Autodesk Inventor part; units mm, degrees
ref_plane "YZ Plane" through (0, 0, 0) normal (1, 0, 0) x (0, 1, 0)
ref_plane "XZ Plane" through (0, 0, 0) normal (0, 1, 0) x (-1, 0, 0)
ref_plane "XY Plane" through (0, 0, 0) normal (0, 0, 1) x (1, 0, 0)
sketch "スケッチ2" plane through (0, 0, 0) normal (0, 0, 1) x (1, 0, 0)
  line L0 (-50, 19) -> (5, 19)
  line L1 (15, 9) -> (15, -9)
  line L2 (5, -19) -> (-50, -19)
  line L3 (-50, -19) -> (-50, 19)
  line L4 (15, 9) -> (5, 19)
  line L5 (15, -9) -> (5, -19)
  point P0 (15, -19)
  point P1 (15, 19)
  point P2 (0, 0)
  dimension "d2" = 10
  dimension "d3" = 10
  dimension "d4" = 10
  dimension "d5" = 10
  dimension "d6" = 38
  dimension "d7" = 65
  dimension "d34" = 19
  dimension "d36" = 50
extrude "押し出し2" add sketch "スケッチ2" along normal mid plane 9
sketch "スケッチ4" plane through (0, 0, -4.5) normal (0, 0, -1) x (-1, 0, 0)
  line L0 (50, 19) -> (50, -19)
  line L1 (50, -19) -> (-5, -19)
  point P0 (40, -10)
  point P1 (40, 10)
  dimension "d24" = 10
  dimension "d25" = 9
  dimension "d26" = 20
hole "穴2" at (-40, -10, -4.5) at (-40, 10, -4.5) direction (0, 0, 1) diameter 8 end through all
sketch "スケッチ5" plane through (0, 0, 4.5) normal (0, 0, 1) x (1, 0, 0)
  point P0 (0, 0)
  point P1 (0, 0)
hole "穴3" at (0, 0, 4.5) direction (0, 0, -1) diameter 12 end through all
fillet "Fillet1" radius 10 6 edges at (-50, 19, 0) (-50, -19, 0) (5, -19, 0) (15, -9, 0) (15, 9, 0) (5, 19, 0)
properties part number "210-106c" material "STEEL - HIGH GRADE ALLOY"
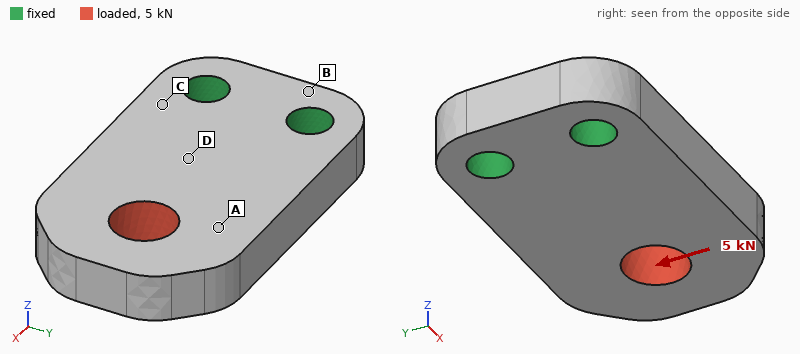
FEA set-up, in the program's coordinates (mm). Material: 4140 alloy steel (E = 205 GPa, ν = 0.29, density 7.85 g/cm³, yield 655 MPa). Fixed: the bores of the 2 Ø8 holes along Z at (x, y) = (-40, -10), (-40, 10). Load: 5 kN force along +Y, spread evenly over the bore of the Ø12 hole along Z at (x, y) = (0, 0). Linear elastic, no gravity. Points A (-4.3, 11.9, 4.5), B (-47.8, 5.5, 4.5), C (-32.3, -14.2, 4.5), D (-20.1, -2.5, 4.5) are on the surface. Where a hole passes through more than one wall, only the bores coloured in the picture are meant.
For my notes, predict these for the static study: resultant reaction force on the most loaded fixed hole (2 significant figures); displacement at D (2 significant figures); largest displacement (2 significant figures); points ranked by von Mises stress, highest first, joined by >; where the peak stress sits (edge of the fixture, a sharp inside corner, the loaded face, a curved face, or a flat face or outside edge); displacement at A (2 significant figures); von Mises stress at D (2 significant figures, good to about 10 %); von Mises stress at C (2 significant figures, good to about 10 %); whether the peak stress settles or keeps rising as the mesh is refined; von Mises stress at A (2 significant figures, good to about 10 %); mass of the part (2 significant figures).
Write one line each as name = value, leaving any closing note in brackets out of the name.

resultant reaction force on the most loaded fixed hole = 8.0 kN
displacement at D = 7.7 µm
largest displacement = 31 µm
points ranked by von Mises stress, highest first, joined by > = C > D > A > B
where the peak stress sits = edge of the fixture
displacement at A = 19 µm
von Mises stress at D = 43 MPa
von Mises stress at C = 56 MPa
whether the peak stress settles or keeps rising as the mesh is refined = keeps rising
von Mises stress at A = 29 MPa
mass of the part = 150 g
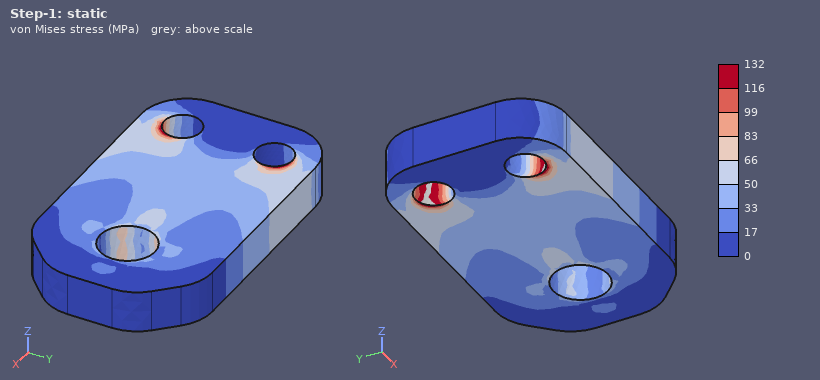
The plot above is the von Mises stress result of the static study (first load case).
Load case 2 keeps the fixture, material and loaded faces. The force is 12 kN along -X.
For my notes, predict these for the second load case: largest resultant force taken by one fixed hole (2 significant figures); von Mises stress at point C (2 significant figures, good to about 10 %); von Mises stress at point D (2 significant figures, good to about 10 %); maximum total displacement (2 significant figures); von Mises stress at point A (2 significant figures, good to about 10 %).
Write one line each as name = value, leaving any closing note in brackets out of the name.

largest resultant force taken by one fixed hole = 6.0 kN
von Mises stress at point C = 35 MPa
von Mises stress at point D = 38 MPa
maximum total displacement = 11 µm
von Mises stress at point A = 38 MPa
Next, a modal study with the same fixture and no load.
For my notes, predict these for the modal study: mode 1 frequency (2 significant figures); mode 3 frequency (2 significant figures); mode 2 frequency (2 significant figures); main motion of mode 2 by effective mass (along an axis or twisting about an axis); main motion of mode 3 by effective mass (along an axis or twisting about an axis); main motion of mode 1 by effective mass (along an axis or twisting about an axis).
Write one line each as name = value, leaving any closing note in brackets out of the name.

mode 1 frequency = 3000 Hz
mode 3 frequency = 8900 Hz
mode 2 frequency = 8300 Hz
main motion of mode 2 by effective mass = twisting about X
main motion of mode 3 by effective mass = along Y
main motion of mode 1 by effective mass = along Z
